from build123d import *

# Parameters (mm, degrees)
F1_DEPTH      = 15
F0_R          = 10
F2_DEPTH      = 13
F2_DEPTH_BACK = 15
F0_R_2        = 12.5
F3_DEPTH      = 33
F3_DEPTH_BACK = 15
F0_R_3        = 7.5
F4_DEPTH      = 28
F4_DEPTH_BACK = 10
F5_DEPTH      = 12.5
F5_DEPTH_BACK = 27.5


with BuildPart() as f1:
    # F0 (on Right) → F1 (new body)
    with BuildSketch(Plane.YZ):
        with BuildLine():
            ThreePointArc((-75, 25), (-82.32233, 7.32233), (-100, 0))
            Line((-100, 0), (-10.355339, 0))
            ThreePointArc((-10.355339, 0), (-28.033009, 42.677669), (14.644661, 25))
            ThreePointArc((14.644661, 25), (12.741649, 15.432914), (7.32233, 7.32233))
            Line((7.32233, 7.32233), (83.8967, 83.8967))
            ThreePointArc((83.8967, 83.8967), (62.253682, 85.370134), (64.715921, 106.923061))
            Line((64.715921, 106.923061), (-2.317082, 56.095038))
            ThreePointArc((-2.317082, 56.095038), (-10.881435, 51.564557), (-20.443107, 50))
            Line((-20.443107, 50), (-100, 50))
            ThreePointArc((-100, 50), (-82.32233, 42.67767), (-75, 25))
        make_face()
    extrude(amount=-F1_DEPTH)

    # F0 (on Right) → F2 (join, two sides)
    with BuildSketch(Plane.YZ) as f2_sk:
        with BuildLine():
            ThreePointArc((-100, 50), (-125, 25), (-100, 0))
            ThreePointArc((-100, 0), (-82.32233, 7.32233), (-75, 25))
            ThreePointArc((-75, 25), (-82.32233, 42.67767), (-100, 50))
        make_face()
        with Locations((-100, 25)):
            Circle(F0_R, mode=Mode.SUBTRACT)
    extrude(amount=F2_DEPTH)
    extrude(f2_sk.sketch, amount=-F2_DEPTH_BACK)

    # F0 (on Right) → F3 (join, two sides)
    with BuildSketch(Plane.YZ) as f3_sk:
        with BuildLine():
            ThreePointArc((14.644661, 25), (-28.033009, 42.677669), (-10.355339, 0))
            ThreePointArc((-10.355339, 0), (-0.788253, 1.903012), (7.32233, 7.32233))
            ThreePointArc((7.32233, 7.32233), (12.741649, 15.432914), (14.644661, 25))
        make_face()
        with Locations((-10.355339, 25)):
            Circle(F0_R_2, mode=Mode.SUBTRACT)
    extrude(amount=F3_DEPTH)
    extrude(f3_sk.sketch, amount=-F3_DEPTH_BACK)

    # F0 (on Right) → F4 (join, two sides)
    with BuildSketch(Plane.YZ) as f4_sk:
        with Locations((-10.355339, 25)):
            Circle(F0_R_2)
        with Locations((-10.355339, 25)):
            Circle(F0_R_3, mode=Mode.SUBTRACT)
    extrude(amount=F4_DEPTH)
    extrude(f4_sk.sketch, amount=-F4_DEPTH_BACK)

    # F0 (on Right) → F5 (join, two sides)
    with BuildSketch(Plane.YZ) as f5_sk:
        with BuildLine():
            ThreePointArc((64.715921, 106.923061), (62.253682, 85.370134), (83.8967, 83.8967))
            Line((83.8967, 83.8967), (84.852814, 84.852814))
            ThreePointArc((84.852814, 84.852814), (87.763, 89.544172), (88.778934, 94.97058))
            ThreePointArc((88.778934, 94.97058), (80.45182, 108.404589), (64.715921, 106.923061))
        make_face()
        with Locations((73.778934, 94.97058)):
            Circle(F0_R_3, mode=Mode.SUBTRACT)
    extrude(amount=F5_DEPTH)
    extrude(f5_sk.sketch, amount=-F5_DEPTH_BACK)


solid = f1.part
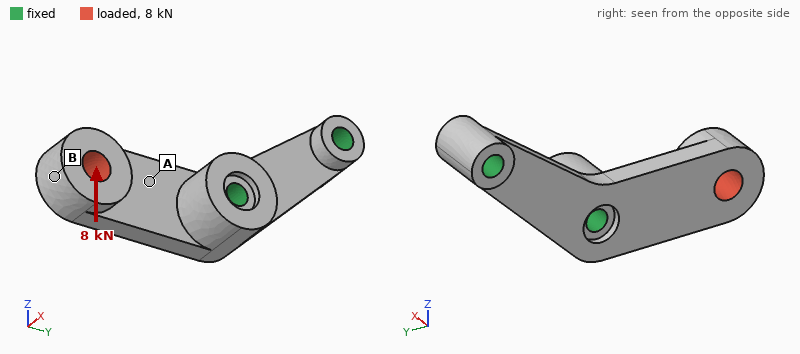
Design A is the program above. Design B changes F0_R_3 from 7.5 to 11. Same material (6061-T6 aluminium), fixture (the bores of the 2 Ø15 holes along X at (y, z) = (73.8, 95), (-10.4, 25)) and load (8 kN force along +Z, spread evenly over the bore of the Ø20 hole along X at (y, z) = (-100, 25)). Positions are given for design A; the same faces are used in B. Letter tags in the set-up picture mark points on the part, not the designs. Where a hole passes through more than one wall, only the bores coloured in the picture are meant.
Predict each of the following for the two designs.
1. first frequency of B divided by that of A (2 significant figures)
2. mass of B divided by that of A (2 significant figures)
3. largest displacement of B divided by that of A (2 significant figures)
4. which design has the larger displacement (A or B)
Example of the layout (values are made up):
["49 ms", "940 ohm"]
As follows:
["1.0", "0.93", "0.86", "A"]
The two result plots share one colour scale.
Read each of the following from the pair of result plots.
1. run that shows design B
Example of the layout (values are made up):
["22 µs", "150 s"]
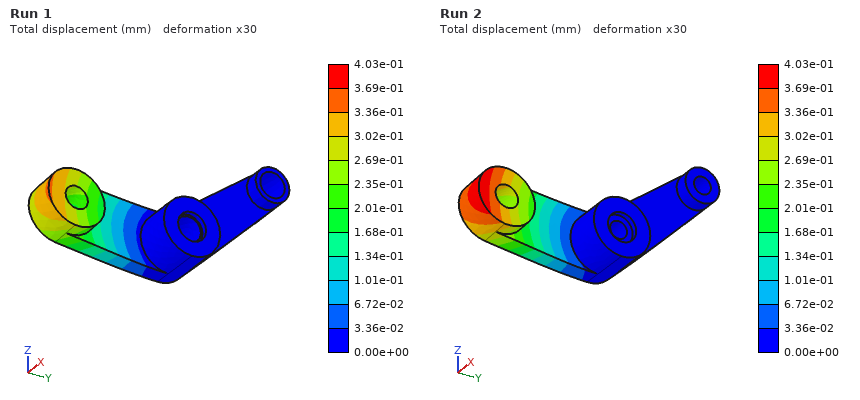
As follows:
["Run 1"]
